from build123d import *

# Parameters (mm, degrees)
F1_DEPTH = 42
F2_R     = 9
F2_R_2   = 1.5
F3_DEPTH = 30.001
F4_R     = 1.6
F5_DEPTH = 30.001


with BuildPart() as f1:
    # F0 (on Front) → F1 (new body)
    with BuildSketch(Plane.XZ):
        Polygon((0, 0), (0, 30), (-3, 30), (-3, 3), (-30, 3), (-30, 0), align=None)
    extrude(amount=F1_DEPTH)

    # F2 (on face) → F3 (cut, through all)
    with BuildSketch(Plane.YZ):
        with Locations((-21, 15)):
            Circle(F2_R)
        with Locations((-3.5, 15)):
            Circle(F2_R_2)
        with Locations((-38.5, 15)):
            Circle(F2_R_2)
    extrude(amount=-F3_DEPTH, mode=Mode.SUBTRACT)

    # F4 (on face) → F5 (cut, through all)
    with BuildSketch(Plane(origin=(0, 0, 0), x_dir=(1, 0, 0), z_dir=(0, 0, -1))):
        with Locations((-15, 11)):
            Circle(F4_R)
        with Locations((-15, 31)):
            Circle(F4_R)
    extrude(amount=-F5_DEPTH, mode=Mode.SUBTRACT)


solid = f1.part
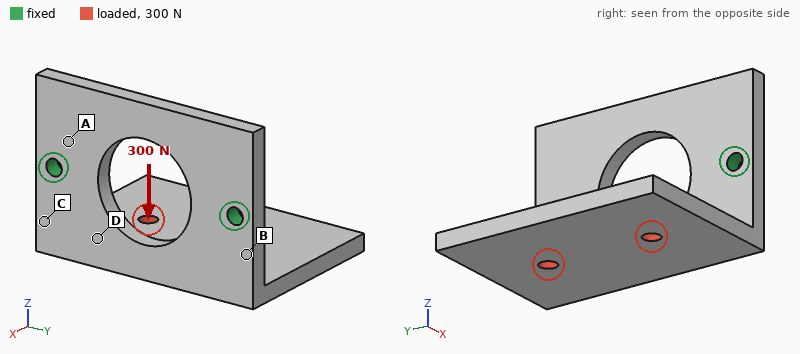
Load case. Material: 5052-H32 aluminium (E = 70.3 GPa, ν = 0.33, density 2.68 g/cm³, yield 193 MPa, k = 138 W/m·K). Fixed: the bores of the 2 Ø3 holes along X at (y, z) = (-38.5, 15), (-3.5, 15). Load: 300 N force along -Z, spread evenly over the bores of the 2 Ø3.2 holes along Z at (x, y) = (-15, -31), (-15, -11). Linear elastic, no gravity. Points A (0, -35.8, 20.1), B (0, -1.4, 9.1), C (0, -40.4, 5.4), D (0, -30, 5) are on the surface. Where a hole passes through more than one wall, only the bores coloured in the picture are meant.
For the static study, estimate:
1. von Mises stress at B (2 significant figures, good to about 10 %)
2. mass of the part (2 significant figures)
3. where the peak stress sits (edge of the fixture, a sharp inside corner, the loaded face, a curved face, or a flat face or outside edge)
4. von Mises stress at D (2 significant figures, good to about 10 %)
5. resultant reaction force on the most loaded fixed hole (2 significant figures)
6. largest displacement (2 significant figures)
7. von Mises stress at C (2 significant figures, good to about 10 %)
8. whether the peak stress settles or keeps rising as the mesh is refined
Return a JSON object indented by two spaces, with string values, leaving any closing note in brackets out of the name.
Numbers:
{
  "von Mises stress at B": "100 MPa",
  "mass of the part": "17 g",
  "where the peak stress sits": "edge of the fixture",
  "von Mises stress at D": "70 MPa",
  "resultant reaction force on the most loaded fixed hole": "160 N",
  "largest displacement": "0.43 mm",
  "von Mises stress at C": "82 MPa",
  "whether the peak stress settles or keeps rising as the mesh is refined": "keeps rising"
}
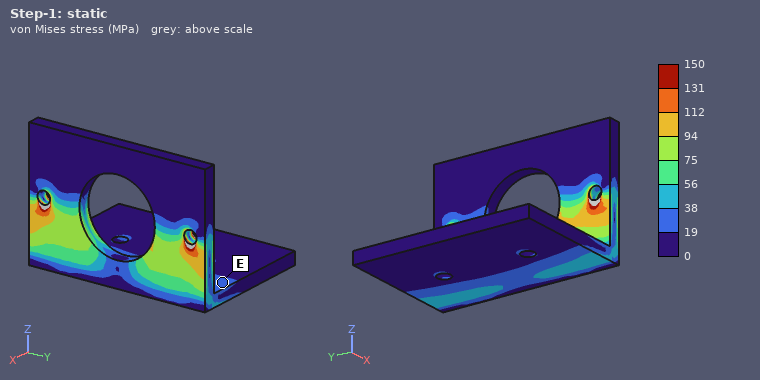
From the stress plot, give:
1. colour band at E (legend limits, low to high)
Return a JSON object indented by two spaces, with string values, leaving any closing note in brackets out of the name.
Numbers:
{
  "colour band at E": "19 to 38 MPa"
}
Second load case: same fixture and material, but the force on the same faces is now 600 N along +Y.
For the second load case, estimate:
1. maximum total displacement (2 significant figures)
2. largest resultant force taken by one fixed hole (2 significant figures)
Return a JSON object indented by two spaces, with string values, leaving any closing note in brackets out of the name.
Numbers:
{
  "maximum total displacement": "0.12 mm",
  "largest resultant force taken by one fixed hole": "430 N"
}
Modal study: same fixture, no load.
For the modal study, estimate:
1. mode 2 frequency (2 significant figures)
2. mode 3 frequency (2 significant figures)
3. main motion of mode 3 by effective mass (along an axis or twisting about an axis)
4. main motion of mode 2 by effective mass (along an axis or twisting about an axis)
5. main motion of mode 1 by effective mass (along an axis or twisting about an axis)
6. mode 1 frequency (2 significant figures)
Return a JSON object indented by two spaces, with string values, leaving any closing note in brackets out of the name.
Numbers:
{
  "mode 2 frequency": "3600 Hz",
  "mode 3 frequency": "5200 Hz",
  "main motion of mode 3 by effective mass": "along X",
  "main motion of mode 2 by effective mass": "along Y",
  "main motion of mode 1 by effective mass": "along Z",
  "mode 1 frequency": "1500 Hz"
}
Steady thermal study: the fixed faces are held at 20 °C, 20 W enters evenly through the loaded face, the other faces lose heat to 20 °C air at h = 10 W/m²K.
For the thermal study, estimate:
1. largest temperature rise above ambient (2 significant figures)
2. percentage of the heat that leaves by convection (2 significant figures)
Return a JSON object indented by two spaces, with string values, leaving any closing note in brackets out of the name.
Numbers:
{
  "largest temperature rise above ambient": "43 K",
  "percentage of the heat that leaves by convection": "5.5 %"
}
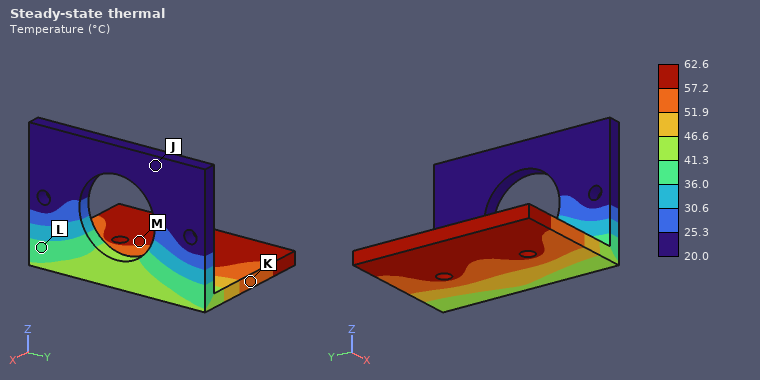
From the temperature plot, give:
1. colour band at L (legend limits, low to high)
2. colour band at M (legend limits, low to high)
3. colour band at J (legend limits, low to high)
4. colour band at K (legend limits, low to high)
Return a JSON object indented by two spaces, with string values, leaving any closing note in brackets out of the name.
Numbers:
{
  "colour band at L": "36.0 to 41.3 °C",
  "colour band at M": "57.2 to 62.6 °C",
  "colour band at J": "20.0 to 25.3 °C",
  "colour band at K": "51.9 to 57.2 °C"
}
